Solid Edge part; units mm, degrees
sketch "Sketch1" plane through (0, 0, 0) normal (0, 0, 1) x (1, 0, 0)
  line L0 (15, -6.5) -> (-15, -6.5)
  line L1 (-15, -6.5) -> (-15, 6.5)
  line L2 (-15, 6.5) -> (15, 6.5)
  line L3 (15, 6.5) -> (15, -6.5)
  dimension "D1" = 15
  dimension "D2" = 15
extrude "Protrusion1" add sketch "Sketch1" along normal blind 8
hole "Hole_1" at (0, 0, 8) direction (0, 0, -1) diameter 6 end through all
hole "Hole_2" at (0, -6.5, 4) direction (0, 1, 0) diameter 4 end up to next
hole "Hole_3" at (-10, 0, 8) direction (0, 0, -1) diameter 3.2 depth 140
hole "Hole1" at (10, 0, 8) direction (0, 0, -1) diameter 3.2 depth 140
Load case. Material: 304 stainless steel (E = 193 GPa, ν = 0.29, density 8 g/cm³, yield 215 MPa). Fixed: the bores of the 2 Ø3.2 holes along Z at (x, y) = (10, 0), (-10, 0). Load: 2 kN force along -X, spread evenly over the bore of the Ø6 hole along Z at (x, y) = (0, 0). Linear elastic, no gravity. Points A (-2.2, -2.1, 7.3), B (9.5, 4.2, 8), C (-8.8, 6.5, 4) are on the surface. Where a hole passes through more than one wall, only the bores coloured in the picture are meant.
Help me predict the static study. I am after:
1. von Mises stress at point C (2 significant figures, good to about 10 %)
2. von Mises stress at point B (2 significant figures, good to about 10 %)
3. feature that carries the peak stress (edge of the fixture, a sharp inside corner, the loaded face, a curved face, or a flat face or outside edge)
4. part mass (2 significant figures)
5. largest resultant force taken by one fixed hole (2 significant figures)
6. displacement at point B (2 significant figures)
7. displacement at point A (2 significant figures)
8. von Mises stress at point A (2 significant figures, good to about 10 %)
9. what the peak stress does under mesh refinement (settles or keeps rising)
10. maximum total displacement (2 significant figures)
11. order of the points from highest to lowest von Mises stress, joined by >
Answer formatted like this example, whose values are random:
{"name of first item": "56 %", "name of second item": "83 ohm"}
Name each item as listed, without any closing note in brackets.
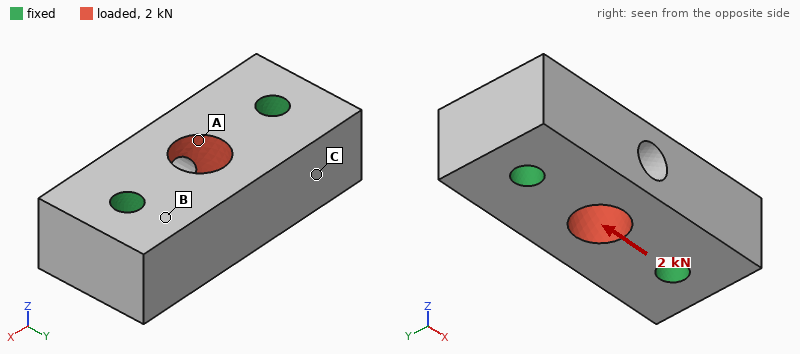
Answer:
{"von Mises stress at point C": "2.8 MPa", "von Mises stress at point B": "5.2 MPa", "feature that carries the peak stress": "edge of the fixture", "part mass": "22 g", "largest resultant force taken by one fixed hole": "1.0 kN", "displacement at point B": "0.27 µm", "displacement at point A": "0.56 µm", "von Mises stress at point A": "20 MPa", "what the peak stress does under mesh refinement": "keeps rising", "maximum total displacement": "0.76 µm", "order of the points from highest to lowest von Mises stress, joined by >": "A > B > C"}
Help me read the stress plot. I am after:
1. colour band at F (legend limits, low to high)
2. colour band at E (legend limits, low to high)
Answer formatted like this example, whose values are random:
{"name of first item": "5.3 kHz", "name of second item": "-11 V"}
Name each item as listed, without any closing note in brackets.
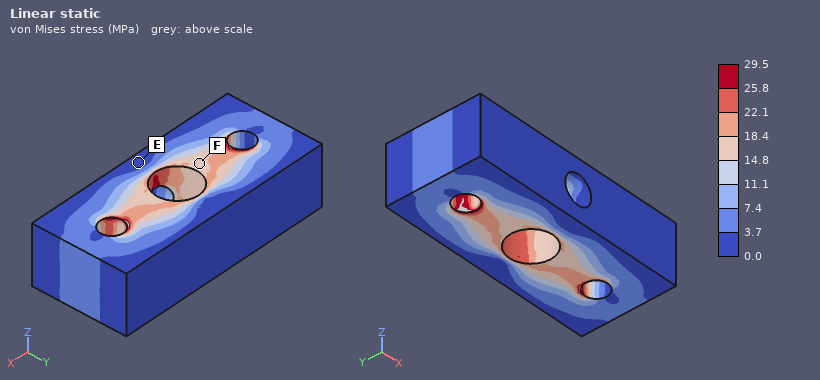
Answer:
{"colour band at F": "14.8 to 18.4 MPa", "colour band at E": "0.0 to 3.7 MPa"}
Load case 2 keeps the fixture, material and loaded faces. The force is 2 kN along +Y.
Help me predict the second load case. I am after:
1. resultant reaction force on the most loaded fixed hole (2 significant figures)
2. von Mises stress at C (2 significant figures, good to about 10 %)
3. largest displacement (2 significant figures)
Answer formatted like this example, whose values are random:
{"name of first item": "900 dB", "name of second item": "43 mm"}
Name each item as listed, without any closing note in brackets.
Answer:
{"resultant reaction force on the most loaded fixed hole": "1.0 kN", "von Mises stress at C": "6.1 MPa", "largest displacement": "2.2 µm"}
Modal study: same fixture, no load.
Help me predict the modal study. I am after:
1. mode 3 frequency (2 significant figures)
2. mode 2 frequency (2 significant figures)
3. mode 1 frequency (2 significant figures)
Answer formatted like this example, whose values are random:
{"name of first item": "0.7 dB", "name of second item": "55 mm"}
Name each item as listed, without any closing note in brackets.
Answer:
{"mode 3 frequency": "61 kHz", "mode 2 frequency": "60 kHz", "mode 1 frequency": "58 kHz"}
